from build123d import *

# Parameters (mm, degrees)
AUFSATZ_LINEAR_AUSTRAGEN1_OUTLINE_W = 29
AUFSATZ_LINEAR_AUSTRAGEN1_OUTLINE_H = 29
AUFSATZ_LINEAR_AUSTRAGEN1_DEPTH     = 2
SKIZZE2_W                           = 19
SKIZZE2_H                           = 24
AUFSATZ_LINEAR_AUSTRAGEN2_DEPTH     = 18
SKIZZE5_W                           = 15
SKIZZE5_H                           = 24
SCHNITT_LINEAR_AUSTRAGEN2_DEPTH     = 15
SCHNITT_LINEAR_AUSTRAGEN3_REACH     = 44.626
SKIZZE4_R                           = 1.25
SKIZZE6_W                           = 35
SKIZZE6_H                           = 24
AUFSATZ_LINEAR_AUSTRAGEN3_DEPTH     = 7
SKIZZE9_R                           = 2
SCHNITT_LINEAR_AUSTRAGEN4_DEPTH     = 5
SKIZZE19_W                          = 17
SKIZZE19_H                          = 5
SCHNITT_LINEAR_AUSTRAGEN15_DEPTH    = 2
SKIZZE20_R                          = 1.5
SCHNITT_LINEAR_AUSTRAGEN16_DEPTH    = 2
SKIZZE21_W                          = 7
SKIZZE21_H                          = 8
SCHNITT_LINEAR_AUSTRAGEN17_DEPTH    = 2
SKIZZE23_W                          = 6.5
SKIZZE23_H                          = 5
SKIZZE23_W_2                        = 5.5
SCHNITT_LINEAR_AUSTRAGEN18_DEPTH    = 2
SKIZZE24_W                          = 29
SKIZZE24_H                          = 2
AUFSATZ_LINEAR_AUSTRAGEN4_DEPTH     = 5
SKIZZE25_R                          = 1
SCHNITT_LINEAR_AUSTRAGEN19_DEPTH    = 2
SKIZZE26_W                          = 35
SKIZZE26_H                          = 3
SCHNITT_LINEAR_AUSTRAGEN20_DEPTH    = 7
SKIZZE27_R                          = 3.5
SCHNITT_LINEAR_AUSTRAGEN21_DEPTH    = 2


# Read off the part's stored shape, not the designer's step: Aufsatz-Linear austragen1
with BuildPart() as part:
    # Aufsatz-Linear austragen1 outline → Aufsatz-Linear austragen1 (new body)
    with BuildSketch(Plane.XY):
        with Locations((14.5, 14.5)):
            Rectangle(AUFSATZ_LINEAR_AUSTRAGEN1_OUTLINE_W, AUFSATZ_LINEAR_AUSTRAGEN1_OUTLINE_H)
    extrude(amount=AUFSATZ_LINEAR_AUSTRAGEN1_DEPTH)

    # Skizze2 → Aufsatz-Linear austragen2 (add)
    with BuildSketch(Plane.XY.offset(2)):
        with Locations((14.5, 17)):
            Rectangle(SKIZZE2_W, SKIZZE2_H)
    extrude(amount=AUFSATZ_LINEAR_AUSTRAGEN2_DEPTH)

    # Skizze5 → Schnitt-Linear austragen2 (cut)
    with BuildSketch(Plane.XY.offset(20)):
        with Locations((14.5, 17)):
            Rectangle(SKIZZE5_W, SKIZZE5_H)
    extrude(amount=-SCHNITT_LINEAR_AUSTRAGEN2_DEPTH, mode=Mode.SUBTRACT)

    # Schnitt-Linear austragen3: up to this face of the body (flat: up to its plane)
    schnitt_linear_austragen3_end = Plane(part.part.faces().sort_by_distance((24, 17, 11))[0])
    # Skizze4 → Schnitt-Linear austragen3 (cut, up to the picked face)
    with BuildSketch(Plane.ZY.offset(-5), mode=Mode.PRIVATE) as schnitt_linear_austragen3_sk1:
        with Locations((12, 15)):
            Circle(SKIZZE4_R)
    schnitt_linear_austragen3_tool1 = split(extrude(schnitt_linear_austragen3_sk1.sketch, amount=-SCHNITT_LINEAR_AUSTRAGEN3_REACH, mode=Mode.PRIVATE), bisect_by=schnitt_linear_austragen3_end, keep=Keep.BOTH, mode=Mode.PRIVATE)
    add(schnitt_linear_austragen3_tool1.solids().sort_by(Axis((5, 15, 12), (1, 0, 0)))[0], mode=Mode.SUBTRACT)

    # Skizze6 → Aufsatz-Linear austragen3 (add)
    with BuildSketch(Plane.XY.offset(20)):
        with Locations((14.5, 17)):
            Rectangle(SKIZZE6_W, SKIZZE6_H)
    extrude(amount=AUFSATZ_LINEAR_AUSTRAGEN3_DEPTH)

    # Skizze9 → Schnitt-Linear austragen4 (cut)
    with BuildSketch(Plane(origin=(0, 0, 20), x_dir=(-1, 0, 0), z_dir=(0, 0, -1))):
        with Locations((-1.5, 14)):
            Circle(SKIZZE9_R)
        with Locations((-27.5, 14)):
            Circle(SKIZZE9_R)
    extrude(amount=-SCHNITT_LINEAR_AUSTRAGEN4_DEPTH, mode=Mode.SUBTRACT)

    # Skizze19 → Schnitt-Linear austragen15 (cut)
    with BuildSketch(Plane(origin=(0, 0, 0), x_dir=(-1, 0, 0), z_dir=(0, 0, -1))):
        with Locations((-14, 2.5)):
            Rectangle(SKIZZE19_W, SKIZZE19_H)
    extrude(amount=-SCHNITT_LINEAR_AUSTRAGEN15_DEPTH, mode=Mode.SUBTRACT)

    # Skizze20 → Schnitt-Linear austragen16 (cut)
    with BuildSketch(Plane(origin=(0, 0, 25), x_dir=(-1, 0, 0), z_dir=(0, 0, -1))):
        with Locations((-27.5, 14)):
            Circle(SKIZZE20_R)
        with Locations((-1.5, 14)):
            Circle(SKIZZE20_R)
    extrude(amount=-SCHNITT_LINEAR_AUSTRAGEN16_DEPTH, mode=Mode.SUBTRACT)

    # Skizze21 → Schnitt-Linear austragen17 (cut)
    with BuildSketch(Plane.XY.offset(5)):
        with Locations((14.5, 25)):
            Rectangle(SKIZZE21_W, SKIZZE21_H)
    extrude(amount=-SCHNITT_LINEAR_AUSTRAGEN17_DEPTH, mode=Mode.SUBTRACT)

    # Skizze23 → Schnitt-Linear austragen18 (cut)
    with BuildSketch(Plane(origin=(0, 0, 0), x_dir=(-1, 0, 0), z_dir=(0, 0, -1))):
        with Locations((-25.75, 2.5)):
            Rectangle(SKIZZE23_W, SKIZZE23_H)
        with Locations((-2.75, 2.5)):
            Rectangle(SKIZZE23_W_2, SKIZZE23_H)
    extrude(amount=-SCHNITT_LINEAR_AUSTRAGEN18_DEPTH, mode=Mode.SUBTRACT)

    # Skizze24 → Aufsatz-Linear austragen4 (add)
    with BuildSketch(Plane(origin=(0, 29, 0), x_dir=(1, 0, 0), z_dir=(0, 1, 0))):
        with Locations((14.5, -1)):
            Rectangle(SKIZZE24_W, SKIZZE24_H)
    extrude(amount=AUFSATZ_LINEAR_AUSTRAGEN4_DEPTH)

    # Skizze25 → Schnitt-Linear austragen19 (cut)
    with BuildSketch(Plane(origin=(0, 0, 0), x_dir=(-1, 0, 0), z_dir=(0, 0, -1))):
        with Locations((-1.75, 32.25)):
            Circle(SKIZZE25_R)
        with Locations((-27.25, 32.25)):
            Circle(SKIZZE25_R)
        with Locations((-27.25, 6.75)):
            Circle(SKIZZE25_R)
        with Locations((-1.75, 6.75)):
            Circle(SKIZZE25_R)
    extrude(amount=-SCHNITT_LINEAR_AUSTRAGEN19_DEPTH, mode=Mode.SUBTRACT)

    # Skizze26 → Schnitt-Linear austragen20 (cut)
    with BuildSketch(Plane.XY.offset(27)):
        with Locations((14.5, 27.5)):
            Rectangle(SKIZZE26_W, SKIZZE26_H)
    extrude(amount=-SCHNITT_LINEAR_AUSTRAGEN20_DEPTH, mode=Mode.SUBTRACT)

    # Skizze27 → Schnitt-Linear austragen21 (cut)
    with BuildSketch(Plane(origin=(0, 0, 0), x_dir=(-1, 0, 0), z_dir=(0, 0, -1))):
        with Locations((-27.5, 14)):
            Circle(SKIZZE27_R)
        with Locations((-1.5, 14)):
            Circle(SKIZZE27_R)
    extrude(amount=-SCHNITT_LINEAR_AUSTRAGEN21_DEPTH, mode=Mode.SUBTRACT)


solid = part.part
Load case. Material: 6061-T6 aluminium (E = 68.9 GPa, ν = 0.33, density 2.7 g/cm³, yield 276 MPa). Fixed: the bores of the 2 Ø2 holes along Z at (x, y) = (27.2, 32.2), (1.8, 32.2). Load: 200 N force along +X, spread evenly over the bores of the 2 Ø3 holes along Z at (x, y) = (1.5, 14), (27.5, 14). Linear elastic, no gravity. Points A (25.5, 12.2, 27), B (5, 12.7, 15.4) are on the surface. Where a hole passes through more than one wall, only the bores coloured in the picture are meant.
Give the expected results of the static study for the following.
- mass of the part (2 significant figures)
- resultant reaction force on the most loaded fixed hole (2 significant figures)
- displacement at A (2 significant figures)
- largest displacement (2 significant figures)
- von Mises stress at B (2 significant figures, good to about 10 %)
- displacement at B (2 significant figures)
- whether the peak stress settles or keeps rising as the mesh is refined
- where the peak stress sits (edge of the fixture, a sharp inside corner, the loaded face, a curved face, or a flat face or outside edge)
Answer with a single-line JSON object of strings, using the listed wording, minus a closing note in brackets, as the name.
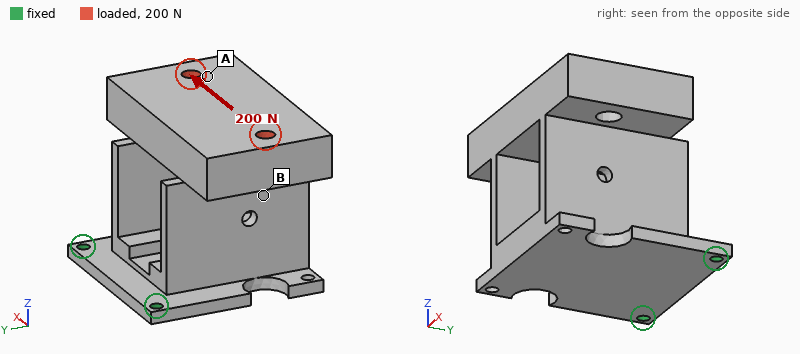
{"mass of the part": "25 g", "resultant reaction force on the most loaded fixed hole": "280 N", "displacement at A": "0.100 mm", "largest displacement": "0.11 mm", "von Mises stress at B": "17 MPa", "displacement at B": "0.065 mm", "whether the peak stress settles or keeps rising as the mesh is refined": "keeps rising", "where the peak stress sits": "edge of the fixture"}
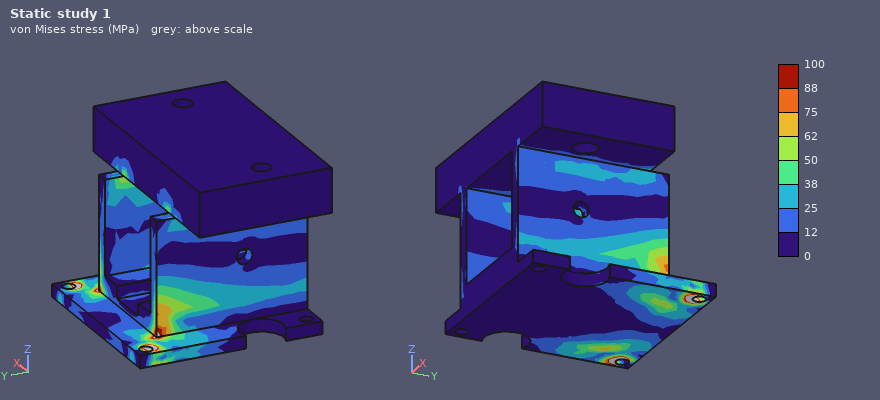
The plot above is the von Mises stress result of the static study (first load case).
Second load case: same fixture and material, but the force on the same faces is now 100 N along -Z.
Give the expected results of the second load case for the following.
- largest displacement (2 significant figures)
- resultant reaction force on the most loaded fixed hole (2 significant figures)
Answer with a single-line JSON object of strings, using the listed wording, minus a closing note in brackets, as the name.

{"largest displacement": "0.38 mm", "resultant reaction force on the most loaded fixed hole": "50 N"}
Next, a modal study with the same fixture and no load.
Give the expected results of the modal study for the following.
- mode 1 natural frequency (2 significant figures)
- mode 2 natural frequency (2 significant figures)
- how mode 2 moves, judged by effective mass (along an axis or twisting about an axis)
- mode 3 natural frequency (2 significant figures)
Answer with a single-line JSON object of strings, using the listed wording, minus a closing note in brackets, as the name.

{"mode 1 natural frequency": "540 Hz", "mode 2 natural frequency": "1900 Hz", "how mode 2 moves, judged by effective mass": "along X", "mode 3 natural frequency": "5200 Hz"}
